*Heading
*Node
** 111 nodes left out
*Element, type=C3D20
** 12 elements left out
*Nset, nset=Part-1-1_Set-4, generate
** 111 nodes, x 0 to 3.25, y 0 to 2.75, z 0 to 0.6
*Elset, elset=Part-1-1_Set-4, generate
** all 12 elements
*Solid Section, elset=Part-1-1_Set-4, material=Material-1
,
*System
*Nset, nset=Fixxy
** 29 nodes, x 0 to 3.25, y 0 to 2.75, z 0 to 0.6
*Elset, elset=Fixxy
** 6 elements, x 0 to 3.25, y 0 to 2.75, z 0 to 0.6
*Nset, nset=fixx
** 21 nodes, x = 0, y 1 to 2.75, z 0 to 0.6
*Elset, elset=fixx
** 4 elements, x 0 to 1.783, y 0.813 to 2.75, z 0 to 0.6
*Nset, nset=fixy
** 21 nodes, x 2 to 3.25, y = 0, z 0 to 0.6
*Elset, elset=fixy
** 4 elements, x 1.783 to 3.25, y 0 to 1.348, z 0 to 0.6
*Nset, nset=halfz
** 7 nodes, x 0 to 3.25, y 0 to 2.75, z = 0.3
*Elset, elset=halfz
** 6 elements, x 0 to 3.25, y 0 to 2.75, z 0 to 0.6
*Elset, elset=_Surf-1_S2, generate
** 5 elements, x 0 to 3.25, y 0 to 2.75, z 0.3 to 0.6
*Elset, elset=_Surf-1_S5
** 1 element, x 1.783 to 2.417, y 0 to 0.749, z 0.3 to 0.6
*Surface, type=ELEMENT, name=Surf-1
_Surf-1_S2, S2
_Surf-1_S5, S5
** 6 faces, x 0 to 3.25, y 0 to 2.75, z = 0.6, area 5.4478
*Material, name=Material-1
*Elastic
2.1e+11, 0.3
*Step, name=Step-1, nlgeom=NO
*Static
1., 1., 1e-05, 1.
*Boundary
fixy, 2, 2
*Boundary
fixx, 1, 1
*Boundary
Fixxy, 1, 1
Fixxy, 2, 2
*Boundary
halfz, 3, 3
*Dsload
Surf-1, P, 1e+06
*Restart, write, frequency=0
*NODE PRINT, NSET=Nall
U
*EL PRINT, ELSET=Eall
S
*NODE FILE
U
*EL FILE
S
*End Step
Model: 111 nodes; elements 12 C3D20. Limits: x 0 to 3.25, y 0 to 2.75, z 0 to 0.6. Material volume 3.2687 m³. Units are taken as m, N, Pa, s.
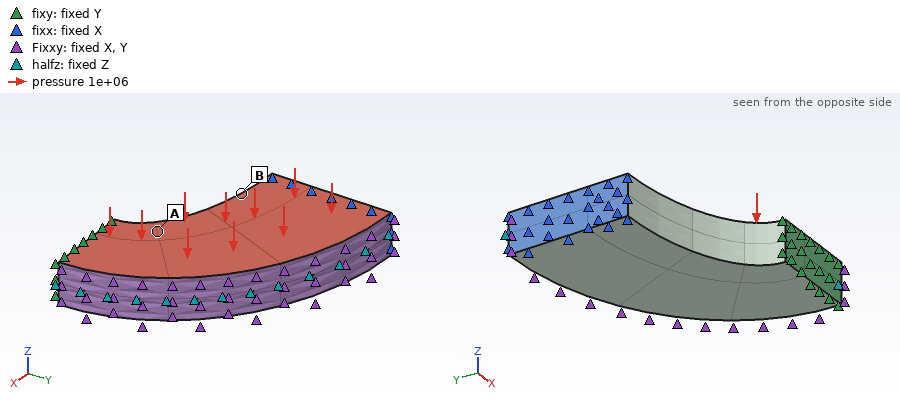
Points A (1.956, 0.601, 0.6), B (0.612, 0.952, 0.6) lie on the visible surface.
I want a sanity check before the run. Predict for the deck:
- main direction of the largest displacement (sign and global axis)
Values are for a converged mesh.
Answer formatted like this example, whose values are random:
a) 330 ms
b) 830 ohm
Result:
a) -Z
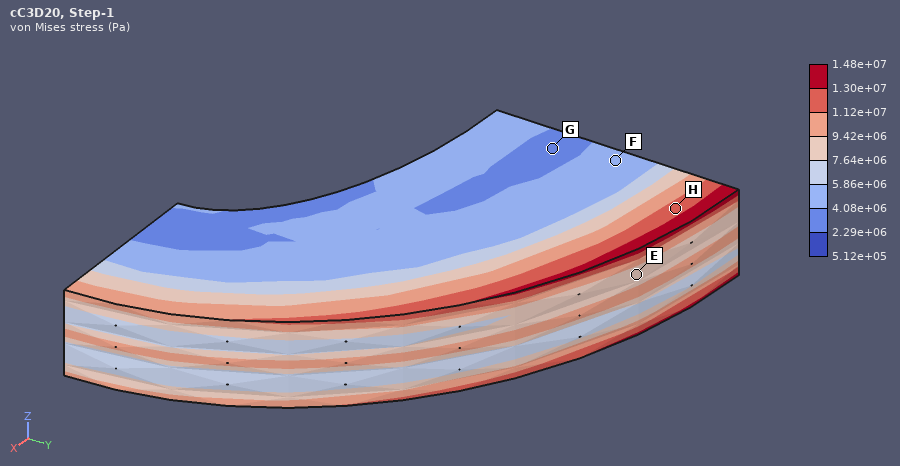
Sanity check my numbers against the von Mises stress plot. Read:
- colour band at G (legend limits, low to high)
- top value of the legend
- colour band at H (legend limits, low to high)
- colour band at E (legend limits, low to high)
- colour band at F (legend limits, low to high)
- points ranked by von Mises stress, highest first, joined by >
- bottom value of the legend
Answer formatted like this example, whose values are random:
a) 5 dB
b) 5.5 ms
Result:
a) 2.29e+06 to 4.08e+06 Pa
b) 1.48e+07 Pa
c) 1.12e+07 to 1.30e+07 Pa
d) 7.64e+06 to 9.42e+06 Pa
e) 4.08e+06 to 5.86e+06 Pa
f) H > E > F > G
g) 5.12e+05 Pa
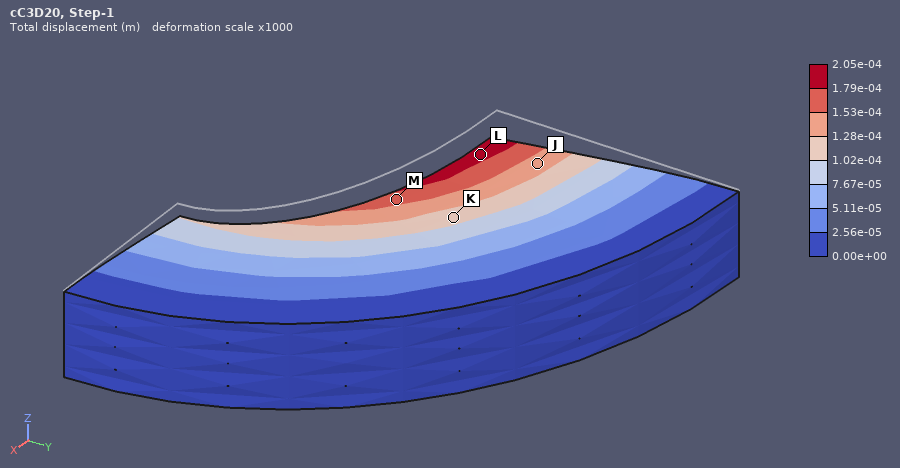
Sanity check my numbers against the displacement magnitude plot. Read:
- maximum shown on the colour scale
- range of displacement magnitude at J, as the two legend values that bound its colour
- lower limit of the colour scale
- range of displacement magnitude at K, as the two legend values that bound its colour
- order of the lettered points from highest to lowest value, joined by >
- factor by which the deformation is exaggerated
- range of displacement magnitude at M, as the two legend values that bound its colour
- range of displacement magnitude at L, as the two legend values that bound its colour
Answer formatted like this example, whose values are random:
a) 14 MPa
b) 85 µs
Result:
a) 2.05e-04 m
b) 1.28e-04 to 1.53e-04 m
c) 0.00e+00 m
d) 1.02e-04 to 1.28e-04 m
e) L > M > J > K
f) 1000
g) 1.53e-04 to 1.79e-04 m
h) 1.79e-04 to 2.05e-04 m
